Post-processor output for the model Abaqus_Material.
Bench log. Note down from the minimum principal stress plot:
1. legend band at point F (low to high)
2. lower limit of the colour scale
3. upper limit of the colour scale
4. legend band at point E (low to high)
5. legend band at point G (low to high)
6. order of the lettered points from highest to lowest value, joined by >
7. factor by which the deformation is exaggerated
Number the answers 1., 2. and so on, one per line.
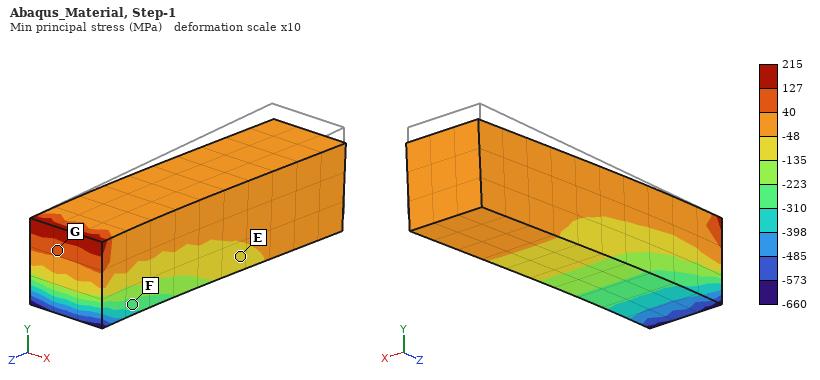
1. -310 to -223 MPa
2. -660 MPa
3. 215 MPa
4. -135 to -48 MPa
5. 40 to 127 MPa
6. G > E > F
7. 10
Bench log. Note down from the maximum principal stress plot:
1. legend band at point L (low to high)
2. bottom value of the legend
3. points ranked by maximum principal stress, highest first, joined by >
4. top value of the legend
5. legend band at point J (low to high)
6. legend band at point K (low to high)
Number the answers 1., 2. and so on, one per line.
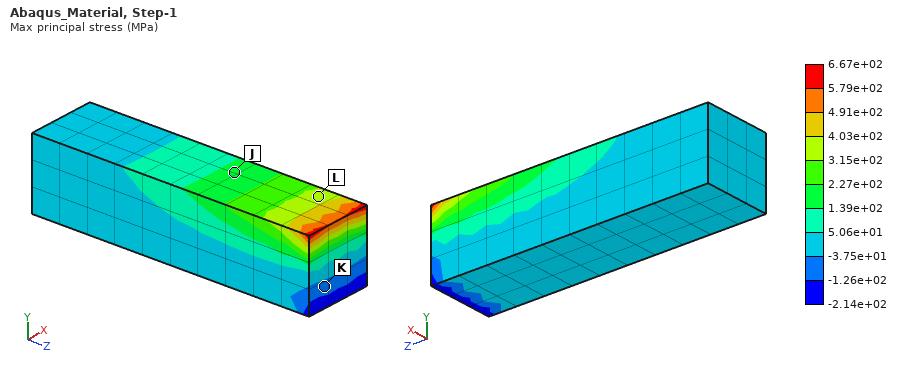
1. 3.15e+02 to 4.03e+02 MPa
2. -2.14e+02 MPa
3. L > J > K
4. 6.67e+02 MPa
5. 1.39e+02 to 2.27e+02 MPa
6. -1.26e+02 to -3.75e+01 MPa
